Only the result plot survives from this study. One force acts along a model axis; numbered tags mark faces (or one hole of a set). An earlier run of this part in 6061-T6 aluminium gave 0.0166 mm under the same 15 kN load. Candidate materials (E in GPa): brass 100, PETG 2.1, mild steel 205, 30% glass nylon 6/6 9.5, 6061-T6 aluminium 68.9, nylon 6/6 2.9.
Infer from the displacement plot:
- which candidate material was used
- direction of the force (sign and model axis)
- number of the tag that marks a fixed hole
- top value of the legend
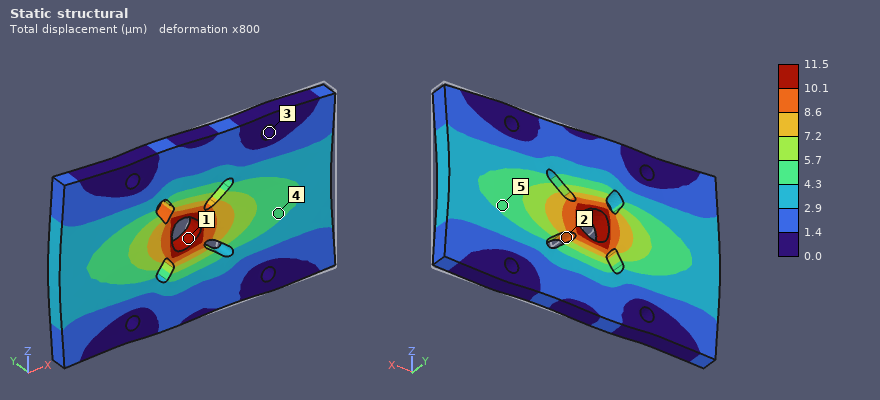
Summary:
brass
-X
3
11.5 µm
